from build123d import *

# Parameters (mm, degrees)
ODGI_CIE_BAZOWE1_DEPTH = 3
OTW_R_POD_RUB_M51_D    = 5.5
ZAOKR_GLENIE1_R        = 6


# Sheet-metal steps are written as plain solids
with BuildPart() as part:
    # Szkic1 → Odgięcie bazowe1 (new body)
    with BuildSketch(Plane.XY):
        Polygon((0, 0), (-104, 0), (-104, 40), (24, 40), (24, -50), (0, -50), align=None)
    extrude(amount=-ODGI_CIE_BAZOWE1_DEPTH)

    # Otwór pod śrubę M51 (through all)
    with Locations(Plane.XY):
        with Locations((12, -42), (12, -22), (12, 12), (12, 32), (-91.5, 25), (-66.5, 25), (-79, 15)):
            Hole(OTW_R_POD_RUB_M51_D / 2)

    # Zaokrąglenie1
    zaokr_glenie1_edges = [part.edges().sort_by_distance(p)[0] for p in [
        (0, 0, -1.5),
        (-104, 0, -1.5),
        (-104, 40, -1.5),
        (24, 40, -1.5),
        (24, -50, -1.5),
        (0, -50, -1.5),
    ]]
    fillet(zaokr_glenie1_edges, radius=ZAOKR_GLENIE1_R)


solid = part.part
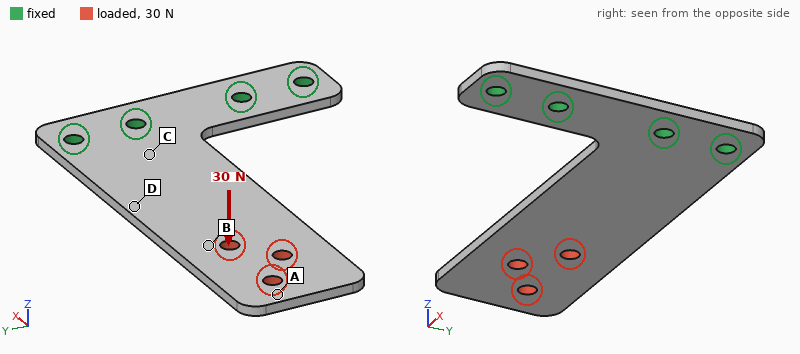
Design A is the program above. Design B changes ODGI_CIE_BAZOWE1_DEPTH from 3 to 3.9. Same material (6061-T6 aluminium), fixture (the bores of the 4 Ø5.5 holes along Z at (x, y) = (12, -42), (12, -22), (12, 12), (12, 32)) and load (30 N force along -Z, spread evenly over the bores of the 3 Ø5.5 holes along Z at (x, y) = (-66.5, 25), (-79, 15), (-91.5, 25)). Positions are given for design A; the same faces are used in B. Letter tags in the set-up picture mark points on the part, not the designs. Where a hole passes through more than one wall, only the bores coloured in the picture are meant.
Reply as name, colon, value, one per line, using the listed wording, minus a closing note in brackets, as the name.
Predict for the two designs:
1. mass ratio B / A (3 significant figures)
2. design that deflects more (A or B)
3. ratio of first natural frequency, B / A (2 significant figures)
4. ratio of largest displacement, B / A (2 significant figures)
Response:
mass ratio B / A: 1.30
design that deflects more: A
ratio of first natural frequency, B / A: 1.3
ratio of largest displacement, B / A: 0.46
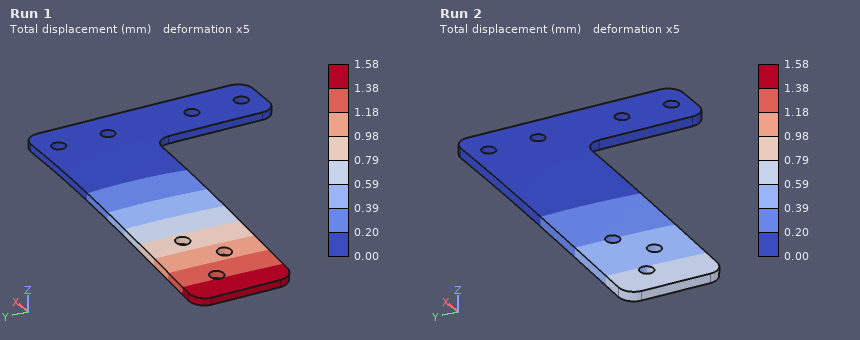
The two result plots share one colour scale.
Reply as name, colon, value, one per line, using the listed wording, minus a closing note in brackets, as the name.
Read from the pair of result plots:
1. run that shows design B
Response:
run that shows design B: Run 2
